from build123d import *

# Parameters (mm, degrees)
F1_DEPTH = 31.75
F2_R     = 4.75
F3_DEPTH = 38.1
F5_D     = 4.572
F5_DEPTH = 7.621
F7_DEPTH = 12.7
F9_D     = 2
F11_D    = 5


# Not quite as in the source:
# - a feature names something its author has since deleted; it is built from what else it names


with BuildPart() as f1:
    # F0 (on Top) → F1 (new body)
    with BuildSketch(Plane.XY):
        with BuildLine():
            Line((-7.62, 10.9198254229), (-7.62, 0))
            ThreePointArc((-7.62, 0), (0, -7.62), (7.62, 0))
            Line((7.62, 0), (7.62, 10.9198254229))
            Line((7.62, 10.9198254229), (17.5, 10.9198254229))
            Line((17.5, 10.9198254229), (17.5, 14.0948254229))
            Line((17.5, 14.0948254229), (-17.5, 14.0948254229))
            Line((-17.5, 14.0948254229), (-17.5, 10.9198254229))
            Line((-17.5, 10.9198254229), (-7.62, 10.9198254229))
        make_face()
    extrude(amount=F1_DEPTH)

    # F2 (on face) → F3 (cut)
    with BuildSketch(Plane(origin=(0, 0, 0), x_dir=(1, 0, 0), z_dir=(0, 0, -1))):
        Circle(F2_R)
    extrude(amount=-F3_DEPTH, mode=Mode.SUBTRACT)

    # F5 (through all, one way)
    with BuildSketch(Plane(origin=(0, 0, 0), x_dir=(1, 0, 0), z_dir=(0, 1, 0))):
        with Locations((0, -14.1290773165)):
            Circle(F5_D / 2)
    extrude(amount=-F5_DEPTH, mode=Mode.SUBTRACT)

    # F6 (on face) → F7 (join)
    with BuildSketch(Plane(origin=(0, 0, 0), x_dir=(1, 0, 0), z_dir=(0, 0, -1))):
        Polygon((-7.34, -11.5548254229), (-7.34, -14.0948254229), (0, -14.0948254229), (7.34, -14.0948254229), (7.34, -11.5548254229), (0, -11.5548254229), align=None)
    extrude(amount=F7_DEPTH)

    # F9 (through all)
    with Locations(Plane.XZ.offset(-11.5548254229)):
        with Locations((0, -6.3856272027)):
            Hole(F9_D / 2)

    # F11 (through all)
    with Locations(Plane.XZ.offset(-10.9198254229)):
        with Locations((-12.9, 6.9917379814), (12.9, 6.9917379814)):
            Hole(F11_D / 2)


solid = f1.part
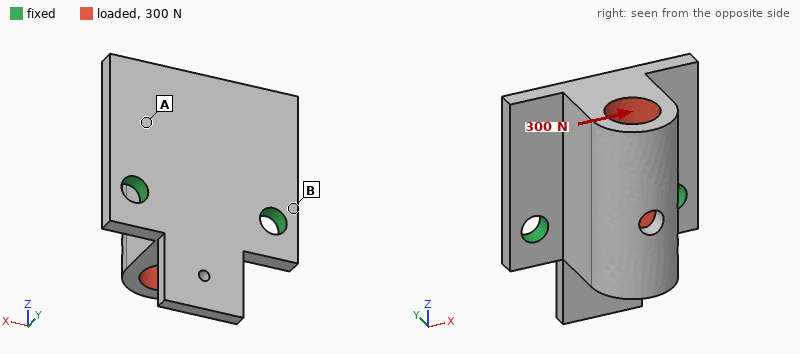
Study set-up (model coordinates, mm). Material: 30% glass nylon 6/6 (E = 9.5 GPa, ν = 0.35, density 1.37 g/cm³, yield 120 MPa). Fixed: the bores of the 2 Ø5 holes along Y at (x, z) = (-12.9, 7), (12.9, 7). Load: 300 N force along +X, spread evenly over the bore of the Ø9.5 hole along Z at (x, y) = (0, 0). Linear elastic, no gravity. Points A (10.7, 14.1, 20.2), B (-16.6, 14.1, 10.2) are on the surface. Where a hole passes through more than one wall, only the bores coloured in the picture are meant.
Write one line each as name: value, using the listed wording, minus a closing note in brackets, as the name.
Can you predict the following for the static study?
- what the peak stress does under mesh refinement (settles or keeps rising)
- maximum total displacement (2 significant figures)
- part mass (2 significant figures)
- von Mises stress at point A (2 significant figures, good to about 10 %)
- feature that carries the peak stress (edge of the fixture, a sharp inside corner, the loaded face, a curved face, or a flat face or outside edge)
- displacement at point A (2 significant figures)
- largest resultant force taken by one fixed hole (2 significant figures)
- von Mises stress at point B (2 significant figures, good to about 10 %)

what the peak stress does under mesh refinement: keeps rising
maximum total displacement: 57 µm
part mass: 13 g
von Mises stress at point A: 3.2 MPa
feature that carries the peak stress: edge of the fixture
displacement at point A: 18 µm
largest resultant force taken by one fixed hole: 260 N
von Mises stress at point B: 7.5 MPa
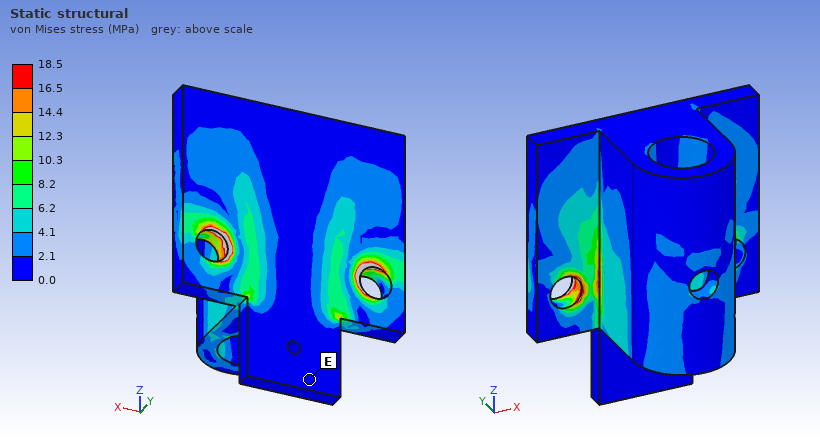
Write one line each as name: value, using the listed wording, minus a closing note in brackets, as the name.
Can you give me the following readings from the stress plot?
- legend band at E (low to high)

legend band at E: 0.0 to 2.1 MPa
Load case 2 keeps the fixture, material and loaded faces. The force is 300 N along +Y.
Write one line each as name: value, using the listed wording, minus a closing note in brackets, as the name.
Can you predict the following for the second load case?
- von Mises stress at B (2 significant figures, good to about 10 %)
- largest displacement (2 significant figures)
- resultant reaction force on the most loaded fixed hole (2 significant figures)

von Mises stress at B: 19 MPa
largest displacement: 0.23 mm
resultant reaction force on the most loaded fixed hole: 160 N
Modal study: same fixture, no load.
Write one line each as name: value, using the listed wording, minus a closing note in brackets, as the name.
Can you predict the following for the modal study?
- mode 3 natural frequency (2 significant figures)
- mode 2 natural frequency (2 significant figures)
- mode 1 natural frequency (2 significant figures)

mode 3 natural frequency: 5400 Hz
mode 2 natural frequency: 5300 Hz
mode 1 natural frequency: 1800 Hz
